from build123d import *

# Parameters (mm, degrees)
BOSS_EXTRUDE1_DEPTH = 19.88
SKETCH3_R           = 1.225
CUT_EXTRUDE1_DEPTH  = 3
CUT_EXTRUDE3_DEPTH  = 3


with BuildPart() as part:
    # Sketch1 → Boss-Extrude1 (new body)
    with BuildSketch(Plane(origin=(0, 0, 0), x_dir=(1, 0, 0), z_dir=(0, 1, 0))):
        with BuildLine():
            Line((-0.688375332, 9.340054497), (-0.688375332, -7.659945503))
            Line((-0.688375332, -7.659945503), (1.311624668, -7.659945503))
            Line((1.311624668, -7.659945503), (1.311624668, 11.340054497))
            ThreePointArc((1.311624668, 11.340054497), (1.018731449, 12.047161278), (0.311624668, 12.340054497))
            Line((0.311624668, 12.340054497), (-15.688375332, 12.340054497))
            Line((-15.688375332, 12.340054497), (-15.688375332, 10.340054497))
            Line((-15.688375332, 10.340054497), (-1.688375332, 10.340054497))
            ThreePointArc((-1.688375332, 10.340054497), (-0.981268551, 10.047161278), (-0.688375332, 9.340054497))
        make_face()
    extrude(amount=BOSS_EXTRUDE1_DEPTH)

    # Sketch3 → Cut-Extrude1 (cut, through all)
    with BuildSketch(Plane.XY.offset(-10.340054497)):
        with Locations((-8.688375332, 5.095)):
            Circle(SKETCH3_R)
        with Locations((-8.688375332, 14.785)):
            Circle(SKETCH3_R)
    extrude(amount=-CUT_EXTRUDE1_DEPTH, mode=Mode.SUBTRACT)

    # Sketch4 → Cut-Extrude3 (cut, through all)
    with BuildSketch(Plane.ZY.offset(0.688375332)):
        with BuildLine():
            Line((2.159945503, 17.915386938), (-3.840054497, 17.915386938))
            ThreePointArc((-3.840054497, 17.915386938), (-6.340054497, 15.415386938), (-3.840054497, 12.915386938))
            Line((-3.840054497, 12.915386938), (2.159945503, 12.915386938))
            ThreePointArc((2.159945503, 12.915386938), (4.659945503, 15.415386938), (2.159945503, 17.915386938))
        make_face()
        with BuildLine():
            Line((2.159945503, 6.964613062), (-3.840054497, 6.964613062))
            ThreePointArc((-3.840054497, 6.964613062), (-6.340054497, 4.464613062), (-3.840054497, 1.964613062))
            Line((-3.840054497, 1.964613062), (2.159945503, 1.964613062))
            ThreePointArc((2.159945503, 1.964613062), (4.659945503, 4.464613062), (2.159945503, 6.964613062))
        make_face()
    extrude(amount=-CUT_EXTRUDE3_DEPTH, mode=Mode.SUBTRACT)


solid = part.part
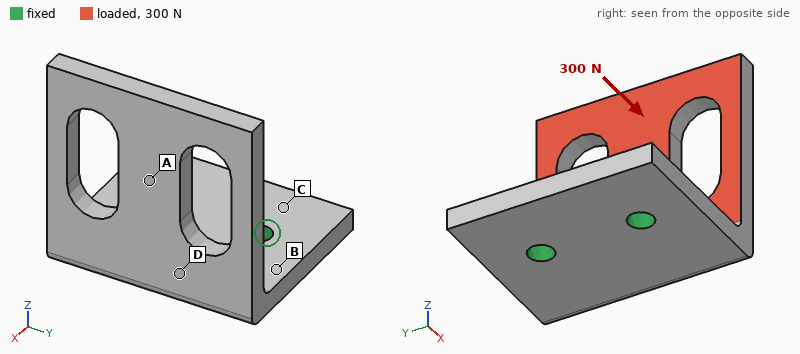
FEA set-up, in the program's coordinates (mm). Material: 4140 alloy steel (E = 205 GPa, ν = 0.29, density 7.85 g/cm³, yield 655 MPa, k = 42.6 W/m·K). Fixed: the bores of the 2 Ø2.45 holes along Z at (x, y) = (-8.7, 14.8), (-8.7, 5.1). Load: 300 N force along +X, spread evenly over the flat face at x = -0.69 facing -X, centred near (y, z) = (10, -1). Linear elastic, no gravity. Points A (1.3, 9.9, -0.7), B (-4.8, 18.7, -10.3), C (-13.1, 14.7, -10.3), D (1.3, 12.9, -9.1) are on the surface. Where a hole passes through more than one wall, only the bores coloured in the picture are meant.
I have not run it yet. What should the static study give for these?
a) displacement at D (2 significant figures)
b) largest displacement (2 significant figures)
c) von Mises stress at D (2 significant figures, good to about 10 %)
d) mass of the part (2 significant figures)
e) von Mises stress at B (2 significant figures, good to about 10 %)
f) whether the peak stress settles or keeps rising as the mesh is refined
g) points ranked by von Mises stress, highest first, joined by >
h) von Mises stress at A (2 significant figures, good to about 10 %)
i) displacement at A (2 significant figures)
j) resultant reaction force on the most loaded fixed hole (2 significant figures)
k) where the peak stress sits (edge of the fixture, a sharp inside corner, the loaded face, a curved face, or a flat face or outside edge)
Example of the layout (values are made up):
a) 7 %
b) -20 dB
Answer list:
a) 0.057 mm
b) 0.30 mm
c) 170 MPa
d) 9.2 g
e) 220 MPa
f) keeps rising
g) B > D > A > C
h) 110 MPa
i) 0.15 mm
j) 150 N
k) edge of the fixture
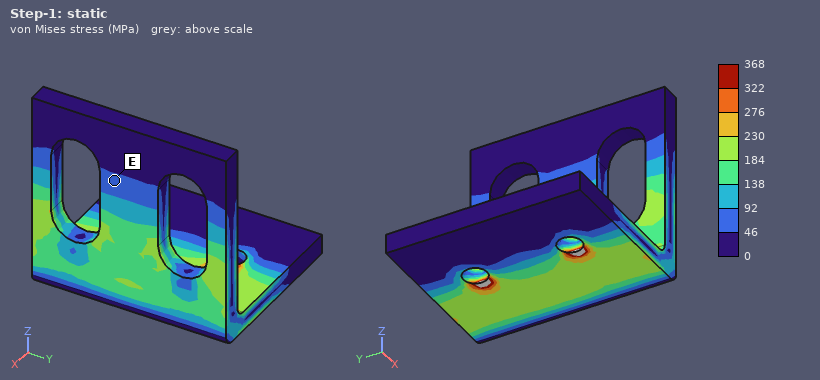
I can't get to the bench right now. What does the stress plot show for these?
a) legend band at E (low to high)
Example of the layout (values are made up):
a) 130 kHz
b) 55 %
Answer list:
a) 46 to 92 MPa
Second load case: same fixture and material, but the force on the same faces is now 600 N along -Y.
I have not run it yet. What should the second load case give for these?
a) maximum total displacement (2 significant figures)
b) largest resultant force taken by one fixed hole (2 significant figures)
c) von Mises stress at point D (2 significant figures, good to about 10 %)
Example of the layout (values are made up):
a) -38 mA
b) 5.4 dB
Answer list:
a) 0.15 mm
b) 700 N
c) 130 MPa
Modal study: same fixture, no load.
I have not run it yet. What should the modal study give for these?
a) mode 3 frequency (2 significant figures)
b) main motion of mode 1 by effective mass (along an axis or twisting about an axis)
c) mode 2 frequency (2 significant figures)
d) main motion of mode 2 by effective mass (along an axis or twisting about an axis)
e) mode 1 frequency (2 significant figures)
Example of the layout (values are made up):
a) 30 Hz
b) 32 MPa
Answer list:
a) 9400 Hz
b) along X
c) 6100 Hz
d) along Y
e) 3000 Hz
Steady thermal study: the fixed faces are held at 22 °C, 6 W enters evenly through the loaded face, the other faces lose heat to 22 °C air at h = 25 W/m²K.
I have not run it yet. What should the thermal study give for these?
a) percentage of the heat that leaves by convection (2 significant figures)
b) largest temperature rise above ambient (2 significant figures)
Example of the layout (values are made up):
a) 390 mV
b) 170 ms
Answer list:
a) 14 %
b) 74 K
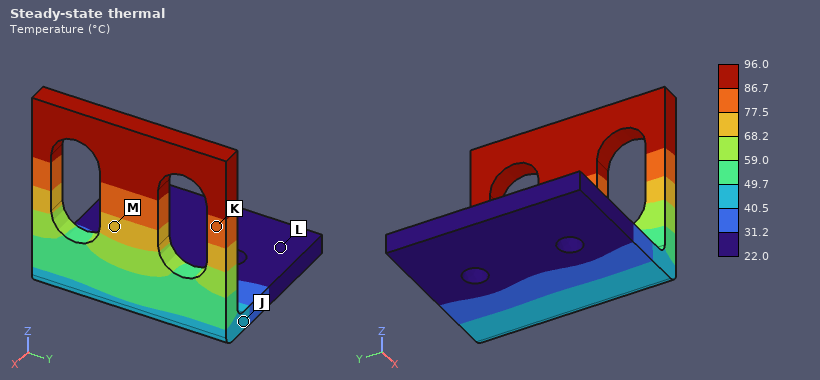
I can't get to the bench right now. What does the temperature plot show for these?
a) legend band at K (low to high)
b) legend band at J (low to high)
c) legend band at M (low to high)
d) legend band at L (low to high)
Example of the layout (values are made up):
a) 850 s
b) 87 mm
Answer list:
a) 77.5 to 86.7 °C
b) 40.5 to 49.7 °C
c) 68.2 to 77.5 °C
d) 22.0 to 31.2 °C
